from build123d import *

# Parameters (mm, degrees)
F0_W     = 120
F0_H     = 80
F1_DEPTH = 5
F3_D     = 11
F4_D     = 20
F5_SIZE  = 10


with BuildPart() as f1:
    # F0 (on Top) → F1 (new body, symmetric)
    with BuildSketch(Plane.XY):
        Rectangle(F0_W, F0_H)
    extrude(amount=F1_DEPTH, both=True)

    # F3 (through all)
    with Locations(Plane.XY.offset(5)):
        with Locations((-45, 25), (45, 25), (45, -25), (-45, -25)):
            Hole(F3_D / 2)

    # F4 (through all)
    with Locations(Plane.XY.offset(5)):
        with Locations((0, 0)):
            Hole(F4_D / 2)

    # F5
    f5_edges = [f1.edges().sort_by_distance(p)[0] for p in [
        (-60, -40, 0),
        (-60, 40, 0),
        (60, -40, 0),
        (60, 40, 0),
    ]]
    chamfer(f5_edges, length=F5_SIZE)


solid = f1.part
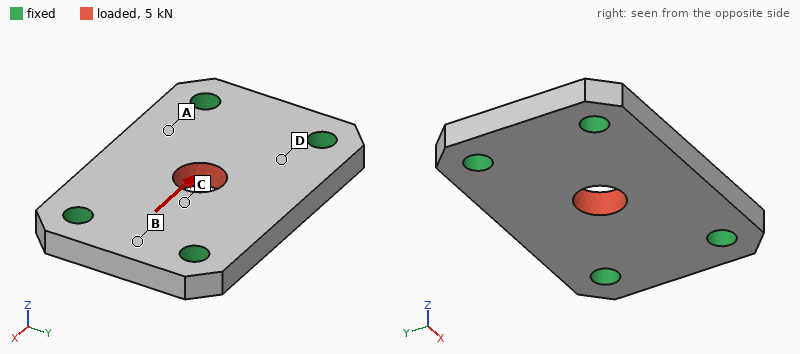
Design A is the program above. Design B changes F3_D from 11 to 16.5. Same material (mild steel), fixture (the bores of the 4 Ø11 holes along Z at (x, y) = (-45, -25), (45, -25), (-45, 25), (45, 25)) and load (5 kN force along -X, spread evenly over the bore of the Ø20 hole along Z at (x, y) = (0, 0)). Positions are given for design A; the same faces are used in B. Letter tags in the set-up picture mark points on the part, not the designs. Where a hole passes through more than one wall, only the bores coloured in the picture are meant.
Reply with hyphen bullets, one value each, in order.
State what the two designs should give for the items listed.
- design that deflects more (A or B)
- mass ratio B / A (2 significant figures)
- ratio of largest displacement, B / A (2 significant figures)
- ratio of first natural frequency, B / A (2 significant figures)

- A
- 0.95
- 0.91
- 1.2
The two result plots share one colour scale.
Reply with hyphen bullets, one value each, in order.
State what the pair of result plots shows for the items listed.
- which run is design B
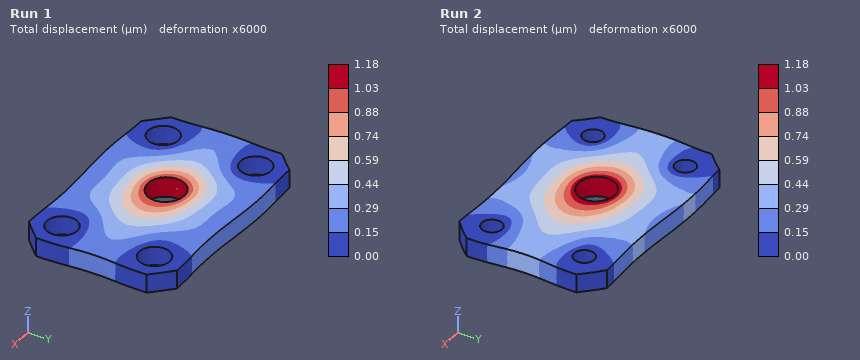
- Run 1
